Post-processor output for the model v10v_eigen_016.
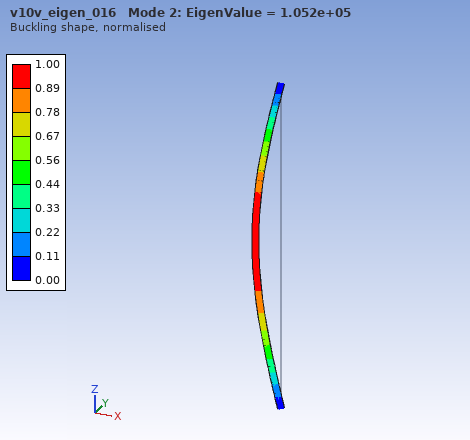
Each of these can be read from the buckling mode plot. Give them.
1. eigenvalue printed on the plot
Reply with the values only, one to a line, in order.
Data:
1.052e+05
